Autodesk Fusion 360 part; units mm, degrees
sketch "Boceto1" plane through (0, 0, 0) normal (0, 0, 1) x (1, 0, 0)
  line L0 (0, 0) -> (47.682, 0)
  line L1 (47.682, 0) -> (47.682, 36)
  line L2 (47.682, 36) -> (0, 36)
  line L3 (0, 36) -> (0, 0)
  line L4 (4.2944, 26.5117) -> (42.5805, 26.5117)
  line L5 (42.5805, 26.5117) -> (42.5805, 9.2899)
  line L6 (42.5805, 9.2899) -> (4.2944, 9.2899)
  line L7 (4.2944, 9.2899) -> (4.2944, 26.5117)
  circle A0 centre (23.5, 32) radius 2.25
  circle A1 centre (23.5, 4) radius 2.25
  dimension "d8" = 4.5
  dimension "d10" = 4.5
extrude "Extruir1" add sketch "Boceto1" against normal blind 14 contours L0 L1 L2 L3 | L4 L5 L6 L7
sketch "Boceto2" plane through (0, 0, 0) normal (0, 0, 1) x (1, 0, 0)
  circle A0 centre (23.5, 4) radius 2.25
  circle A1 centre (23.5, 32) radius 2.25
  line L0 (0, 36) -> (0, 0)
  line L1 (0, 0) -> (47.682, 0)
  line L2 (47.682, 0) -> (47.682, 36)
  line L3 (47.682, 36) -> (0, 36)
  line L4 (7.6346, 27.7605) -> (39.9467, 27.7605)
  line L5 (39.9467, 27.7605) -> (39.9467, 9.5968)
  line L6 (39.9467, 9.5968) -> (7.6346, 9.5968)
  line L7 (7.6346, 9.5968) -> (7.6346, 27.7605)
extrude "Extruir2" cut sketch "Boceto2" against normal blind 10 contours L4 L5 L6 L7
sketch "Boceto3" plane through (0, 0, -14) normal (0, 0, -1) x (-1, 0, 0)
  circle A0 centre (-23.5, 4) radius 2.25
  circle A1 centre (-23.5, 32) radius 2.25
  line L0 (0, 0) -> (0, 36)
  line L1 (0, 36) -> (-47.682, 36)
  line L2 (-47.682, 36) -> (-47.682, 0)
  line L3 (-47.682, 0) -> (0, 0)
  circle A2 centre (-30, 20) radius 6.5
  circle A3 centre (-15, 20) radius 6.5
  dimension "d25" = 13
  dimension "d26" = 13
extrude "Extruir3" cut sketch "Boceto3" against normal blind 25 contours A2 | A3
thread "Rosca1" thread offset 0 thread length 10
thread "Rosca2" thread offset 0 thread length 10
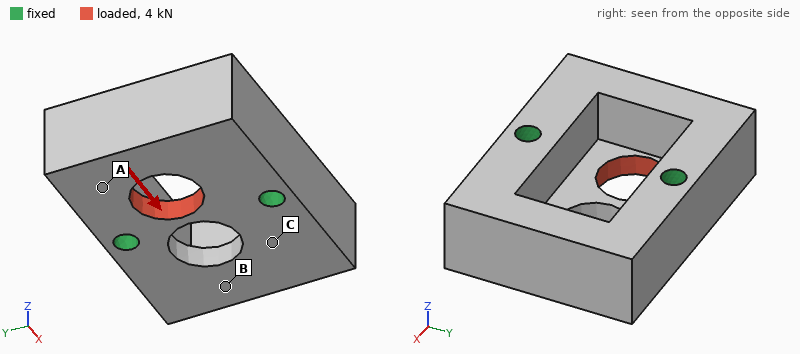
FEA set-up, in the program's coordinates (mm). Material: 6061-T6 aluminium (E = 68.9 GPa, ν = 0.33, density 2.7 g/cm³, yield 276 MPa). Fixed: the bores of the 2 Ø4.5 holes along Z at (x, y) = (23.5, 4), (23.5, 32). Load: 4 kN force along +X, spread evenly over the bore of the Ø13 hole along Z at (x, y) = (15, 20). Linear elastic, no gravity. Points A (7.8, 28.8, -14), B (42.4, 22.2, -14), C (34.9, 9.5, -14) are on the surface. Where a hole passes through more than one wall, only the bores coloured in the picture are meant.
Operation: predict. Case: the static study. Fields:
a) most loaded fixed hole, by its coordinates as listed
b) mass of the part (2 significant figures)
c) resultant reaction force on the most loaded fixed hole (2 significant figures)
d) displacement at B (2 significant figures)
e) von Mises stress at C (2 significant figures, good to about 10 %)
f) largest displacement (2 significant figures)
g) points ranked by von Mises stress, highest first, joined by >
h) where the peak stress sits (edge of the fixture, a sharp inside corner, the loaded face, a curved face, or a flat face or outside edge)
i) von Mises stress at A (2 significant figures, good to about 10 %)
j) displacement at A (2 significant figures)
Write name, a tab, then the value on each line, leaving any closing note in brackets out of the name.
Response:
most loaded fixed hole, by its coordinates as listed	(23.5, 32)
mass of the part	45 g
resultant reaction force on the most loaded fixed hole	2.3 kN
displacement at B	2.3 µm
von Mises stress at C	11 MPa
largest displacement	15 µm
points ranked by von Mises stress, highest first, joined by >	A > C > B
where the peak stress sits	a curved face
von Mises stress at A	21 MPa
displacement at A	8.0 µm
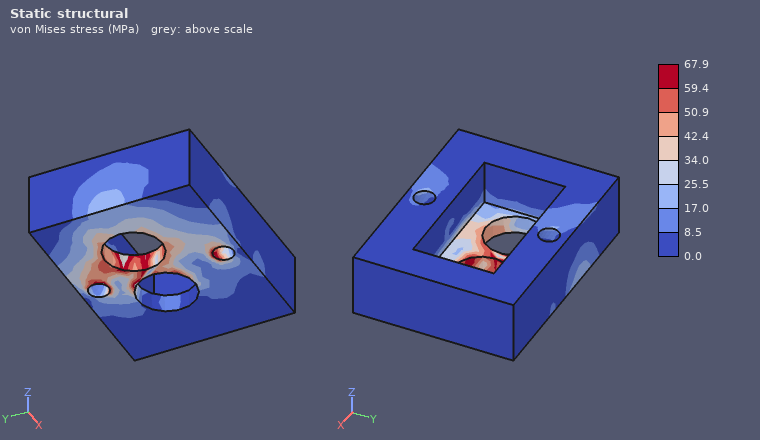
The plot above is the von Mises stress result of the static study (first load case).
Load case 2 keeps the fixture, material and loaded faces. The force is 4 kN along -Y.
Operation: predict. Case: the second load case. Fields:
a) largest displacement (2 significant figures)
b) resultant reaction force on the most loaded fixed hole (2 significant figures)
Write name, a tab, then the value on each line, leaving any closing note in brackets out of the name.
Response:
largest displacement	17 µm
resultant reaction force on the most loaded fixed hole	2.1 kN
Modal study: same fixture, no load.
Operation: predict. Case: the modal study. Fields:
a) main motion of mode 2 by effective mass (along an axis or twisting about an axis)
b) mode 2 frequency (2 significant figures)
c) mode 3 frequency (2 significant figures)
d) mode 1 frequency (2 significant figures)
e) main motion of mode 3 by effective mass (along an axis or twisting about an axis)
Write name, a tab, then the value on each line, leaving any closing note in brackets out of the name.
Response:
main motion of mode 2 by effective mass	along Z
mode 2 frequency	14 kHz
mode 3 frequency	15 kHz
mode 1 frequency	13 kHz
main motion of mode 3 by effective mass	twisting about Z
